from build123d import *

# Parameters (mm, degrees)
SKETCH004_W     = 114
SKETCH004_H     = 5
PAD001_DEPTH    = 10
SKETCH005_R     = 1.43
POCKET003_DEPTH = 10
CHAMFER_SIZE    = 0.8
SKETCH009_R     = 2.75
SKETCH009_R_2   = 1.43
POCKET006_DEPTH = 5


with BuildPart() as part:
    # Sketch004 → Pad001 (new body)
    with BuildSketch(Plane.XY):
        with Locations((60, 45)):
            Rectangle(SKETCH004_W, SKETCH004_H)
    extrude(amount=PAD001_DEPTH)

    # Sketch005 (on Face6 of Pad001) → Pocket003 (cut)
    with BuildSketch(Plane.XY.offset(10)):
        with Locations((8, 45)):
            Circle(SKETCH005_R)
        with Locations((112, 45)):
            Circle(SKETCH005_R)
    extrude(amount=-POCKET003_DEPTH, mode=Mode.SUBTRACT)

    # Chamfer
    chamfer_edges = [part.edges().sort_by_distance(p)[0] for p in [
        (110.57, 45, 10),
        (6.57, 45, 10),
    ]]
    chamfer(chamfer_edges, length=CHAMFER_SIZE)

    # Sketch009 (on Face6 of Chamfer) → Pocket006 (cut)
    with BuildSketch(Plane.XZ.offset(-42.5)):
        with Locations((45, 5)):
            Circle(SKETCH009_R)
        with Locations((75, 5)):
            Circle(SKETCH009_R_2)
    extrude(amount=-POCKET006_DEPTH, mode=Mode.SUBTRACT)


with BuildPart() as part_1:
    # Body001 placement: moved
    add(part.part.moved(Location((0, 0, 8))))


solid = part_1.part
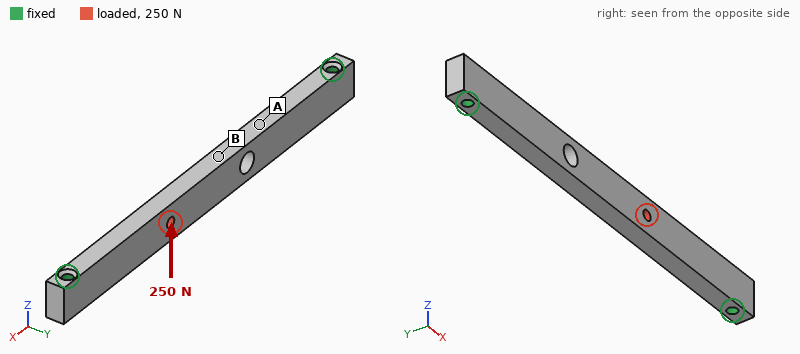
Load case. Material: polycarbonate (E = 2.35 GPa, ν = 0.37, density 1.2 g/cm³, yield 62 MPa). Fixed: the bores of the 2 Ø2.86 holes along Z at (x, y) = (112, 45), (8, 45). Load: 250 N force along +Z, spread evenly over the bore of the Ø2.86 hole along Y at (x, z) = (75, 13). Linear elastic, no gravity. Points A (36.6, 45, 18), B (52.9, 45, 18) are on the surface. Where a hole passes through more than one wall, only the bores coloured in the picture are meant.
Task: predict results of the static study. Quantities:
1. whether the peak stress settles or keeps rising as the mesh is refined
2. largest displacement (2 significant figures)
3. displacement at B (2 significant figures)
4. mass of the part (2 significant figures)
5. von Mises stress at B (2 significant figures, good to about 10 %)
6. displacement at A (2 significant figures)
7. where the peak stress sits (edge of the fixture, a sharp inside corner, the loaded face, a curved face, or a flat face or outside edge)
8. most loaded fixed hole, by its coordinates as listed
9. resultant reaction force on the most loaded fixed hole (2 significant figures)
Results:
keeps rising
1.4 mm
1.2 mm
6.5 g
14 MPa
0.65 mm
edge of the fixture
(112, 45)
180 N
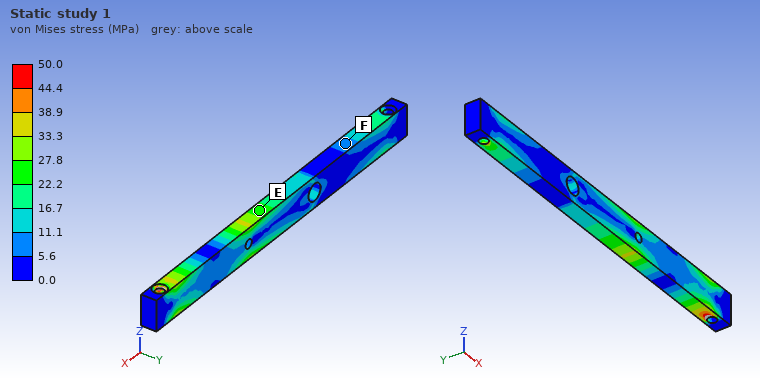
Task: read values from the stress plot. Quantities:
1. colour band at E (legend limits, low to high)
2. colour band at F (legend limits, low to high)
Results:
22.2 to 27.8 MPa
5.6 to 11.1 MPa
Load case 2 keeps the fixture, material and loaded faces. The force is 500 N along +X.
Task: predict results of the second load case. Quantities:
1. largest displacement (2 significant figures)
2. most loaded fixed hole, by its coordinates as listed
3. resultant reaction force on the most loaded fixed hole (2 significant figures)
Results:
0.11 mm
(112, 45)
340 N
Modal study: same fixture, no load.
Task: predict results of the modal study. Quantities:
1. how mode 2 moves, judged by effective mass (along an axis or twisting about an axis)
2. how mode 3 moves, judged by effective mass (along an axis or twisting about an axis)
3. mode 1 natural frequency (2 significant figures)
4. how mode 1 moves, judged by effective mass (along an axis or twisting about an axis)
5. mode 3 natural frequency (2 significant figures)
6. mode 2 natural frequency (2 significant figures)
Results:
along Z
twisting about Z
660 Hz
along Y
1700 Hz
1300 Hz
